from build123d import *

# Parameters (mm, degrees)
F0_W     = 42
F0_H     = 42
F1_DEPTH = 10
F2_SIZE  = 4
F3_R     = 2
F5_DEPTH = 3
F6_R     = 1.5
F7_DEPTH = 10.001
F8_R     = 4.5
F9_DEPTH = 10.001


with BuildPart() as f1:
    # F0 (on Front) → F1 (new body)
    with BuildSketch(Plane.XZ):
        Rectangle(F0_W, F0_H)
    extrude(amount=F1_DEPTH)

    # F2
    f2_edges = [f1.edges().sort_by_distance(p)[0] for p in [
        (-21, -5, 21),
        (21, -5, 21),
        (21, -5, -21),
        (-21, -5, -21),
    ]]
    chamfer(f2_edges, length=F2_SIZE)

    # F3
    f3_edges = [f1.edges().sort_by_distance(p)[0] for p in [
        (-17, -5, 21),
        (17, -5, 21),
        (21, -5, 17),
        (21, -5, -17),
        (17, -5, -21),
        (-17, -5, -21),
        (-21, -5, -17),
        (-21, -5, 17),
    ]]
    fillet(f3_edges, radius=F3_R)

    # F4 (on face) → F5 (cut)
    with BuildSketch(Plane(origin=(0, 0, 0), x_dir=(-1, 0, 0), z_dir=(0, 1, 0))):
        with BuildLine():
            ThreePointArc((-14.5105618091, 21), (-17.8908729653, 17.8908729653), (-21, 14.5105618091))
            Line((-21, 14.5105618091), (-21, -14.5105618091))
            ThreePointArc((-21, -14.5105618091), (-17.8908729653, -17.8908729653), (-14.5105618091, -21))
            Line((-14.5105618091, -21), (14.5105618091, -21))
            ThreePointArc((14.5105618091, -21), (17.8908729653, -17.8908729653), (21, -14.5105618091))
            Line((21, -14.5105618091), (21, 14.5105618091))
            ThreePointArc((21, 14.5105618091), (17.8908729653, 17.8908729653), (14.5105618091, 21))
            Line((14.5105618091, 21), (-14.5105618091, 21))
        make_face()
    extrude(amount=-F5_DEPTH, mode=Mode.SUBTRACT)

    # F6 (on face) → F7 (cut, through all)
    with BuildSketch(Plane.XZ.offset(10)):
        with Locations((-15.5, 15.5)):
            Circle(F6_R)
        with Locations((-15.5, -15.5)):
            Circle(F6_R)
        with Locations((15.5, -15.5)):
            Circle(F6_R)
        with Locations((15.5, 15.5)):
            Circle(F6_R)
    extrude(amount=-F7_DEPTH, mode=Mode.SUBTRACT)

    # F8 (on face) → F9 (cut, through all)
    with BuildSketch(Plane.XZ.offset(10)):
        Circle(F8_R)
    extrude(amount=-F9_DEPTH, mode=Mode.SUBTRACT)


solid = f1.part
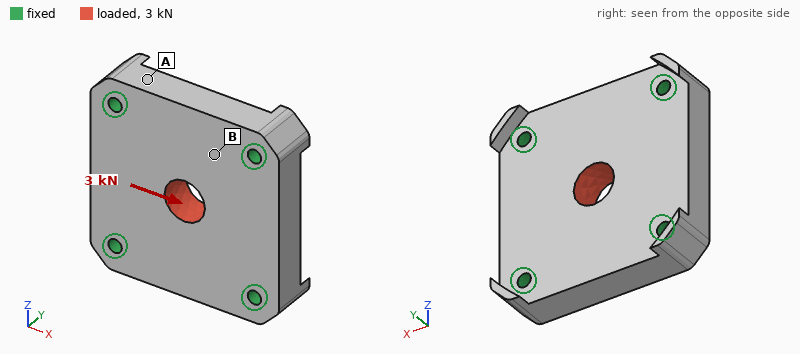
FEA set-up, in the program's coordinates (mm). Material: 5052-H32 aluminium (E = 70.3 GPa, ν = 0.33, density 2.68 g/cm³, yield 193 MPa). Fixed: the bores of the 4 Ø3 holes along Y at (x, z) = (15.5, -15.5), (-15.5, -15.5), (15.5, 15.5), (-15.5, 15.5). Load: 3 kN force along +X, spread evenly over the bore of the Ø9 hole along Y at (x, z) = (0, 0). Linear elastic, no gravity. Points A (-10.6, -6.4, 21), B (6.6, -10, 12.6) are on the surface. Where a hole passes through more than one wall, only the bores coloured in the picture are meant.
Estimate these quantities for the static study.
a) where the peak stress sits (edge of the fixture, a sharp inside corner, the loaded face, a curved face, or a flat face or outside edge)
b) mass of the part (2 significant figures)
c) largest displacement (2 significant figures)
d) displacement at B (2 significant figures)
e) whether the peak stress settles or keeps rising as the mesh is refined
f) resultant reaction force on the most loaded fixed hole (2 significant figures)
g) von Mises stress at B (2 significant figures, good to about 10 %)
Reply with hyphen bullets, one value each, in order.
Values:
- edge of the fixture
- 31 g
- 4.2 µm
- 1.3 µm
- keeps rising
- 820 N
- 8.8 MPa
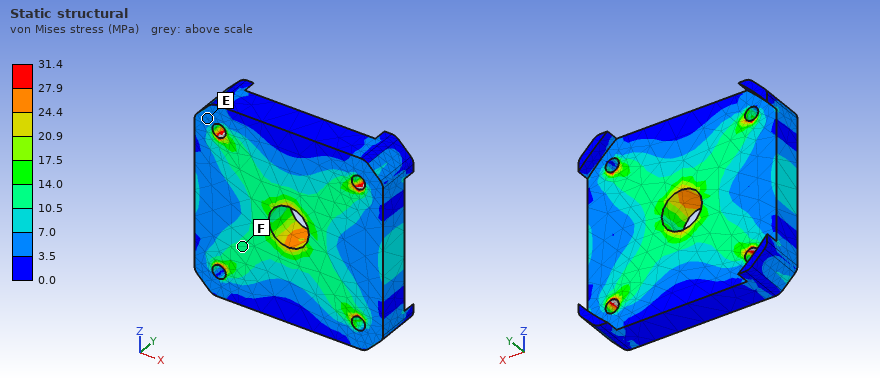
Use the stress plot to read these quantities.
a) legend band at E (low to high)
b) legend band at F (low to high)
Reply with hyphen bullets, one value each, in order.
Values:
- 3.5 to 7.0 MPa
- 10.5 to 14.0 MPa
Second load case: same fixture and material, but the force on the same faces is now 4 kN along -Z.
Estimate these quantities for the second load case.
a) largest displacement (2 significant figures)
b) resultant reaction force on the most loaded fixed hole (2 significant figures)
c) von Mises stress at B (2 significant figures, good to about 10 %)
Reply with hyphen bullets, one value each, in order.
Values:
- 5.6 µm
- 1.1 kN
- 12 MPa
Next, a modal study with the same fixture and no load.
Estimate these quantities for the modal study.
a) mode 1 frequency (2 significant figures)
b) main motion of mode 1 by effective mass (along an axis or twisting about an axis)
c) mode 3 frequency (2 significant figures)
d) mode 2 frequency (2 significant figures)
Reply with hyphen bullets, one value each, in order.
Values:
- 21 kHz
- along Y
- 31 kHz
- 31 kHz
